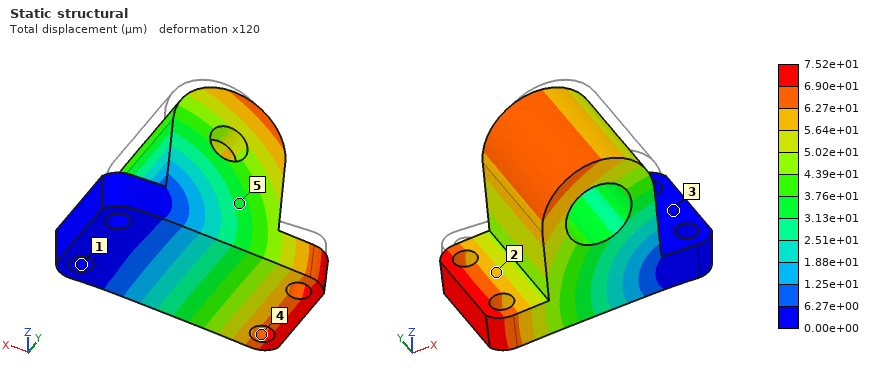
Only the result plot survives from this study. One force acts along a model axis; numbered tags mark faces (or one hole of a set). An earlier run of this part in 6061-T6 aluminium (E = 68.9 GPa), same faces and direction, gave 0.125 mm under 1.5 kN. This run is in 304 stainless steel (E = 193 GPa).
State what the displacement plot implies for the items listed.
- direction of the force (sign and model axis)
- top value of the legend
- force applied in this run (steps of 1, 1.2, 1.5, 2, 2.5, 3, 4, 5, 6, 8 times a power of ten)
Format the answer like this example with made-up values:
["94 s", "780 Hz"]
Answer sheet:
["-Z", "7.52e+01 µm", "2.5 kN"]
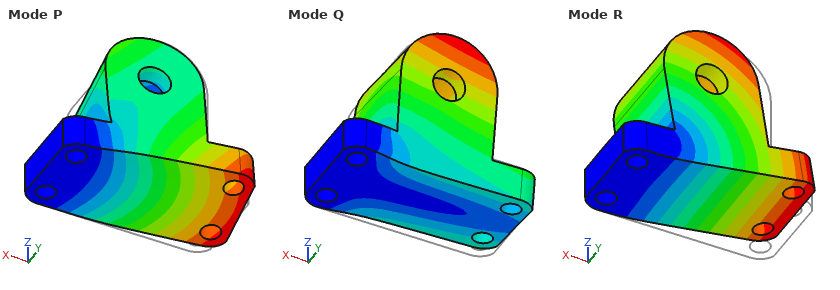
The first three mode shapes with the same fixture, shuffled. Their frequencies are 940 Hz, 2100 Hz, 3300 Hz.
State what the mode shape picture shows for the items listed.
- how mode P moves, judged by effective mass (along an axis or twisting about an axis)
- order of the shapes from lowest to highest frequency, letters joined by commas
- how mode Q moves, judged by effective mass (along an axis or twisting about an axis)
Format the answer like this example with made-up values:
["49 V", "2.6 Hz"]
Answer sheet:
["along Y", "R, Q, P", "along Y"]
